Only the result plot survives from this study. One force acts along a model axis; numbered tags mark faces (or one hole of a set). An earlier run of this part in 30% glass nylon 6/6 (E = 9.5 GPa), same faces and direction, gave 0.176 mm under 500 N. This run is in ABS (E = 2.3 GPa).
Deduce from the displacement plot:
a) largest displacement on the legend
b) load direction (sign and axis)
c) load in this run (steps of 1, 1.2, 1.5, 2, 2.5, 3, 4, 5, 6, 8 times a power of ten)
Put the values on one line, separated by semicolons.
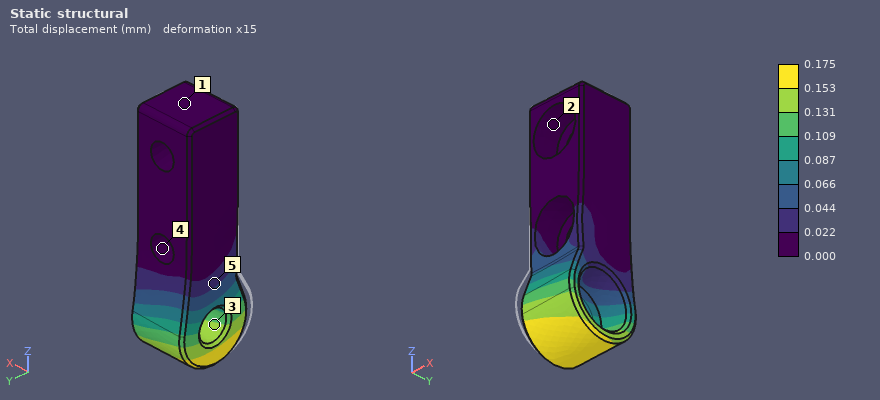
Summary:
0.175 mm; +Y; 120 N
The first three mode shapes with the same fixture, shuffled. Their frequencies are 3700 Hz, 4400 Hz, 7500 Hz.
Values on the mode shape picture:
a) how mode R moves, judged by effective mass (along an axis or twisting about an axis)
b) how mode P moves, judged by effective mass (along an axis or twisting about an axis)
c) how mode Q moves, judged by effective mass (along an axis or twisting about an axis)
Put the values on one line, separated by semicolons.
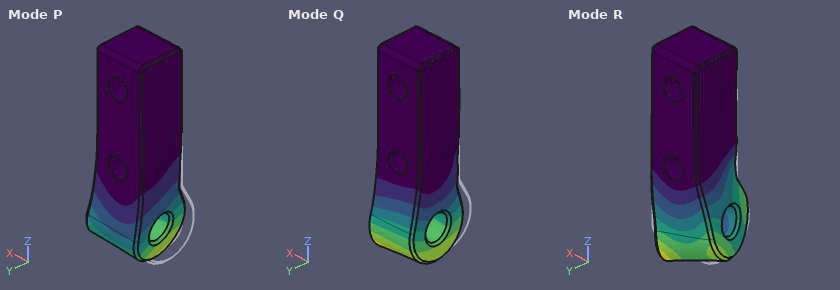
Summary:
twisting about Z; along X; along Y
